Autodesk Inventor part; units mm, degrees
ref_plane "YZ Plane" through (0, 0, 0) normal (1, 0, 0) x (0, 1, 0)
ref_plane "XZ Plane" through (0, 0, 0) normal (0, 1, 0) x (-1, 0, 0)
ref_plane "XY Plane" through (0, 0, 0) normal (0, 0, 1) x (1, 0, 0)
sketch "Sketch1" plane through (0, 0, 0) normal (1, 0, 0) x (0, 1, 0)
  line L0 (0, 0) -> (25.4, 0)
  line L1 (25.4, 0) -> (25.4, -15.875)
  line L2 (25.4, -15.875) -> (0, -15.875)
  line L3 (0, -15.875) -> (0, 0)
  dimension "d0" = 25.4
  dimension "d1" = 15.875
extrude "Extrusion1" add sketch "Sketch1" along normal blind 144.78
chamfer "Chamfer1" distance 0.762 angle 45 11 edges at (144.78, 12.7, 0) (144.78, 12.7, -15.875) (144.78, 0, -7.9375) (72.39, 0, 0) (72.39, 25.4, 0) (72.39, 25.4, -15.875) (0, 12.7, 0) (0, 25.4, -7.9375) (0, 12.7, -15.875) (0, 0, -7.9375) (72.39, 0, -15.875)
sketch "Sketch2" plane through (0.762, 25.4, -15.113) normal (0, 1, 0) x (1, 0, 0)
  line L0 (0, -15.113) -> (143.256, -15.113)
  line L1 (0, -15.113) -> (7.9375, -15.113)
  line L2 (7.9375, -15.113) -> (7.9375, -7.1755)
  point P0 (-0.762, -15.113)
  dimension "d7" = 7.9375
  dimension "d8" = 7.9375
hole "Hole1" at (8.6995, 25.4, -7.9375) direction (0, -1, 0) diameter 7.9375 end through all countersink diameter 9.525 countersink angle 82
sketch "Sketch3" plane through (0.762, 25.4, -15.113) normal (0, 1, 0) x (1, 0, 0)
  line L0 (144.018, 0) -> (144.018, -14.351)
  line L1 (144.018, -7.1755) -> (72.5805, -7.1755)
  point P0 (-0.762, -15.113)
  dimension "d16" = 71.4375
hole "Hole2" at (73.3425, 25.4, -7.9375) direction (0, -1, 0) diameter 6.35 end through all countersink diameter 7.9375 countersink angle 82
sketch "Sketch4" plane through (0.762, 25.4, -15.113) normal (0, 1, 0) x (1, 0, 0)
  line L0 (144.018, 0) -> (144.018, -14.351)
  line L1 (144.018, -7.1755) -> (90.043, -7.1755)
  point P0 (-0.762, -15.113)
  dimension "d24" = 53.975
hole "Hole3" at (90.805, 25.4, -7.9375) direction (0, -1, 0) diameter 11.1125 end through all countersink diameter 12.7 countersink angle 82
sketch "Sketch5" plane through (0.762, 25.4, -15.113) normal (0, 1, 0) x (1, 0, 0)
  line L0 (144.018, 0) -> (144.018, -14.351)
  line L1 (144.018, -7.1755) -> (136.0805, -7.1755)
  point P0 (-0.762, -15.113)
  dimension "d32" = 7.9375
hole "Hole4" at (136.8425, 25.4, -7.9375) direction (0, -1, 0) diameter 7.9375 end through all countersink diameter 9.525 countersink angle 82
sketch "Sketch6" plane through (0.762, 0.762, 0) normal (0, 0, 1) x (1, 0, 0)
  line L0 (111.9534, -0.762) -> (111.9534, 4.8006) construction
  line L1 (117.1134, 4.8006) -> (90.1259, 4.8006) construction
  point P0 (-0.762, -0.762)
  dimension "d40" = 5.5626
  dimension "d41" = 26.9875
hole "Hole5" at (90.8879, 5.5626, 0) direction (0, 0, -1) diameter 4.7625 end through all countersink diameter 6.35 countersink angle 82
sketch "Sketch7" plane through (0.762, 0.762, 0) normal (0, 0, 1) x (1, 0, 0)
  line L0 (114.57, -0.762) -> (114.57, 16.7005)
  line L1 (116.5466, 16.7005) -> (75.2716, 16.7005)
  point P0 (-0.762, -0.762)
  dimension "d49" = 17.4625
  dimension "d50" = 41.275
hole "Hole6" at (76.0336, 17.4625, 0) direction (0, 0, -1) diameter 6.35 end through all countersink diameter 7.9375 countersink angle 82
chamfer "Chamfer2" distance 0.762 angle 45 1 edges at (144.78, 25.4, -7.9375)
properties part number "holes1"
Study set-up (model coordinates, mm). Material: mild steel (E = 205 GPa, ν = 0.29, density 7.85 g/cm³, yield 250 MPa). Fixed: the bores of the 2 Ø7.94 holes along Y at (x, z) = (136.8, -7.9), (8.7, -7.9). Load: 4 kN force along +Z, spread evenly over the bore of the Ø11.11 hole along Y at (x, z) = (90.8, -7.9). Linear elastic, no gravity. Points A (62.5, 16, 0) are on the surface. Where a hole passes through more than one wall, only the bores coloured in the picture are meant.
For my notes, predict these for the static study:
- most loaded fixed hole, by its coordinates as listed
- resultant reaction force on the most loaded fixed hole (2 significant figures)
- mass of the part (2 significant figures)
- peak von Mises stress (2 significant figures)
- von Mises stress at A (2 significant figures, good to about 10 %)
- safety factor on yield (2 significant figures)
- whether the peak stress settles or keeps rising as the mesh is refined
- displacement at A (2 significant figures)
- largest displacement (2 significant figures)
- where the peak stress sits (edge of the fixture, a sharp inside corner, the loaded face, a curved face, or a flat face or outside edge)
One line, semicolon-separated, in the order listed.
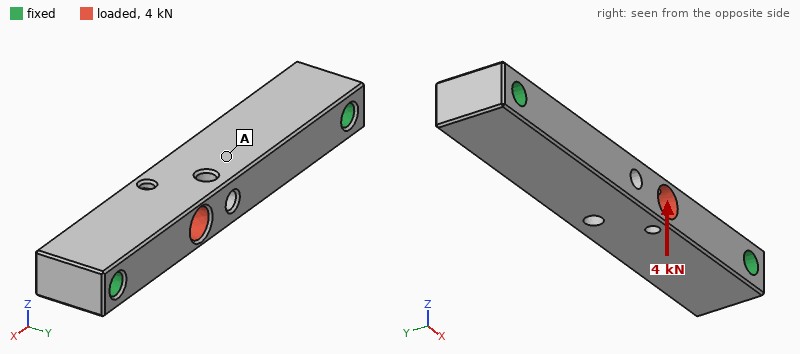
(136.8, -7.9); 2.8 kN; 410 g; 200 MPa; 15 MPa; 1.3; settles; 24 µm; 33 µm; the loaded face
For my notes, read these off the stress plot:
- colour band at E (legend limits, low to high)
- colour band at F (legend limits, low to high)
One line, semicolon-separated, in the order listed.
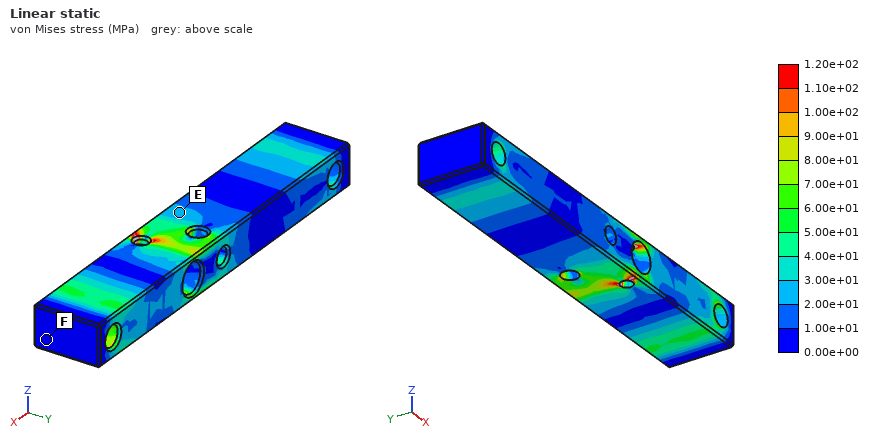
2.00e+01 to 3.00e+01 MPa; 0.00e+00 to 1.00e+01 MPa
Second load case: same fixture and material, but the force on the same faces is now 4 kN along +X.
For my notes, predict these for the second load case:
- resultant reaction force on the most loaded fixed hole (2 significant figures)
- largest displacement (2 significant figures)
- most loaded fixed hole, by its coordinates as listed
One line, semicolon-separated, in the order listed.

2.5 kN; 1.7 µm; (136.8, -7.9)
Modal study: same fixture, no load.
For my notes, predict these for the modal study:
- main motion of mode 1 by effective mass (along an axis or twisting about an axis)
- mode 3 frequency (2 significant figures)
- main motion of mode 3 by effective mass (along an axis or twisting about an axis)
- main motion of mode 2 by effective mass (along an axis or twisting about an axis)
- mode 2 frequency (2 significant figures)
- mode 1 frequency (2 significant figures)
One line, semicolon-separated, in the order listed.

along Z; 11 kHz; twisting about X; along Y; 6900 Hz; 4600 Hz
